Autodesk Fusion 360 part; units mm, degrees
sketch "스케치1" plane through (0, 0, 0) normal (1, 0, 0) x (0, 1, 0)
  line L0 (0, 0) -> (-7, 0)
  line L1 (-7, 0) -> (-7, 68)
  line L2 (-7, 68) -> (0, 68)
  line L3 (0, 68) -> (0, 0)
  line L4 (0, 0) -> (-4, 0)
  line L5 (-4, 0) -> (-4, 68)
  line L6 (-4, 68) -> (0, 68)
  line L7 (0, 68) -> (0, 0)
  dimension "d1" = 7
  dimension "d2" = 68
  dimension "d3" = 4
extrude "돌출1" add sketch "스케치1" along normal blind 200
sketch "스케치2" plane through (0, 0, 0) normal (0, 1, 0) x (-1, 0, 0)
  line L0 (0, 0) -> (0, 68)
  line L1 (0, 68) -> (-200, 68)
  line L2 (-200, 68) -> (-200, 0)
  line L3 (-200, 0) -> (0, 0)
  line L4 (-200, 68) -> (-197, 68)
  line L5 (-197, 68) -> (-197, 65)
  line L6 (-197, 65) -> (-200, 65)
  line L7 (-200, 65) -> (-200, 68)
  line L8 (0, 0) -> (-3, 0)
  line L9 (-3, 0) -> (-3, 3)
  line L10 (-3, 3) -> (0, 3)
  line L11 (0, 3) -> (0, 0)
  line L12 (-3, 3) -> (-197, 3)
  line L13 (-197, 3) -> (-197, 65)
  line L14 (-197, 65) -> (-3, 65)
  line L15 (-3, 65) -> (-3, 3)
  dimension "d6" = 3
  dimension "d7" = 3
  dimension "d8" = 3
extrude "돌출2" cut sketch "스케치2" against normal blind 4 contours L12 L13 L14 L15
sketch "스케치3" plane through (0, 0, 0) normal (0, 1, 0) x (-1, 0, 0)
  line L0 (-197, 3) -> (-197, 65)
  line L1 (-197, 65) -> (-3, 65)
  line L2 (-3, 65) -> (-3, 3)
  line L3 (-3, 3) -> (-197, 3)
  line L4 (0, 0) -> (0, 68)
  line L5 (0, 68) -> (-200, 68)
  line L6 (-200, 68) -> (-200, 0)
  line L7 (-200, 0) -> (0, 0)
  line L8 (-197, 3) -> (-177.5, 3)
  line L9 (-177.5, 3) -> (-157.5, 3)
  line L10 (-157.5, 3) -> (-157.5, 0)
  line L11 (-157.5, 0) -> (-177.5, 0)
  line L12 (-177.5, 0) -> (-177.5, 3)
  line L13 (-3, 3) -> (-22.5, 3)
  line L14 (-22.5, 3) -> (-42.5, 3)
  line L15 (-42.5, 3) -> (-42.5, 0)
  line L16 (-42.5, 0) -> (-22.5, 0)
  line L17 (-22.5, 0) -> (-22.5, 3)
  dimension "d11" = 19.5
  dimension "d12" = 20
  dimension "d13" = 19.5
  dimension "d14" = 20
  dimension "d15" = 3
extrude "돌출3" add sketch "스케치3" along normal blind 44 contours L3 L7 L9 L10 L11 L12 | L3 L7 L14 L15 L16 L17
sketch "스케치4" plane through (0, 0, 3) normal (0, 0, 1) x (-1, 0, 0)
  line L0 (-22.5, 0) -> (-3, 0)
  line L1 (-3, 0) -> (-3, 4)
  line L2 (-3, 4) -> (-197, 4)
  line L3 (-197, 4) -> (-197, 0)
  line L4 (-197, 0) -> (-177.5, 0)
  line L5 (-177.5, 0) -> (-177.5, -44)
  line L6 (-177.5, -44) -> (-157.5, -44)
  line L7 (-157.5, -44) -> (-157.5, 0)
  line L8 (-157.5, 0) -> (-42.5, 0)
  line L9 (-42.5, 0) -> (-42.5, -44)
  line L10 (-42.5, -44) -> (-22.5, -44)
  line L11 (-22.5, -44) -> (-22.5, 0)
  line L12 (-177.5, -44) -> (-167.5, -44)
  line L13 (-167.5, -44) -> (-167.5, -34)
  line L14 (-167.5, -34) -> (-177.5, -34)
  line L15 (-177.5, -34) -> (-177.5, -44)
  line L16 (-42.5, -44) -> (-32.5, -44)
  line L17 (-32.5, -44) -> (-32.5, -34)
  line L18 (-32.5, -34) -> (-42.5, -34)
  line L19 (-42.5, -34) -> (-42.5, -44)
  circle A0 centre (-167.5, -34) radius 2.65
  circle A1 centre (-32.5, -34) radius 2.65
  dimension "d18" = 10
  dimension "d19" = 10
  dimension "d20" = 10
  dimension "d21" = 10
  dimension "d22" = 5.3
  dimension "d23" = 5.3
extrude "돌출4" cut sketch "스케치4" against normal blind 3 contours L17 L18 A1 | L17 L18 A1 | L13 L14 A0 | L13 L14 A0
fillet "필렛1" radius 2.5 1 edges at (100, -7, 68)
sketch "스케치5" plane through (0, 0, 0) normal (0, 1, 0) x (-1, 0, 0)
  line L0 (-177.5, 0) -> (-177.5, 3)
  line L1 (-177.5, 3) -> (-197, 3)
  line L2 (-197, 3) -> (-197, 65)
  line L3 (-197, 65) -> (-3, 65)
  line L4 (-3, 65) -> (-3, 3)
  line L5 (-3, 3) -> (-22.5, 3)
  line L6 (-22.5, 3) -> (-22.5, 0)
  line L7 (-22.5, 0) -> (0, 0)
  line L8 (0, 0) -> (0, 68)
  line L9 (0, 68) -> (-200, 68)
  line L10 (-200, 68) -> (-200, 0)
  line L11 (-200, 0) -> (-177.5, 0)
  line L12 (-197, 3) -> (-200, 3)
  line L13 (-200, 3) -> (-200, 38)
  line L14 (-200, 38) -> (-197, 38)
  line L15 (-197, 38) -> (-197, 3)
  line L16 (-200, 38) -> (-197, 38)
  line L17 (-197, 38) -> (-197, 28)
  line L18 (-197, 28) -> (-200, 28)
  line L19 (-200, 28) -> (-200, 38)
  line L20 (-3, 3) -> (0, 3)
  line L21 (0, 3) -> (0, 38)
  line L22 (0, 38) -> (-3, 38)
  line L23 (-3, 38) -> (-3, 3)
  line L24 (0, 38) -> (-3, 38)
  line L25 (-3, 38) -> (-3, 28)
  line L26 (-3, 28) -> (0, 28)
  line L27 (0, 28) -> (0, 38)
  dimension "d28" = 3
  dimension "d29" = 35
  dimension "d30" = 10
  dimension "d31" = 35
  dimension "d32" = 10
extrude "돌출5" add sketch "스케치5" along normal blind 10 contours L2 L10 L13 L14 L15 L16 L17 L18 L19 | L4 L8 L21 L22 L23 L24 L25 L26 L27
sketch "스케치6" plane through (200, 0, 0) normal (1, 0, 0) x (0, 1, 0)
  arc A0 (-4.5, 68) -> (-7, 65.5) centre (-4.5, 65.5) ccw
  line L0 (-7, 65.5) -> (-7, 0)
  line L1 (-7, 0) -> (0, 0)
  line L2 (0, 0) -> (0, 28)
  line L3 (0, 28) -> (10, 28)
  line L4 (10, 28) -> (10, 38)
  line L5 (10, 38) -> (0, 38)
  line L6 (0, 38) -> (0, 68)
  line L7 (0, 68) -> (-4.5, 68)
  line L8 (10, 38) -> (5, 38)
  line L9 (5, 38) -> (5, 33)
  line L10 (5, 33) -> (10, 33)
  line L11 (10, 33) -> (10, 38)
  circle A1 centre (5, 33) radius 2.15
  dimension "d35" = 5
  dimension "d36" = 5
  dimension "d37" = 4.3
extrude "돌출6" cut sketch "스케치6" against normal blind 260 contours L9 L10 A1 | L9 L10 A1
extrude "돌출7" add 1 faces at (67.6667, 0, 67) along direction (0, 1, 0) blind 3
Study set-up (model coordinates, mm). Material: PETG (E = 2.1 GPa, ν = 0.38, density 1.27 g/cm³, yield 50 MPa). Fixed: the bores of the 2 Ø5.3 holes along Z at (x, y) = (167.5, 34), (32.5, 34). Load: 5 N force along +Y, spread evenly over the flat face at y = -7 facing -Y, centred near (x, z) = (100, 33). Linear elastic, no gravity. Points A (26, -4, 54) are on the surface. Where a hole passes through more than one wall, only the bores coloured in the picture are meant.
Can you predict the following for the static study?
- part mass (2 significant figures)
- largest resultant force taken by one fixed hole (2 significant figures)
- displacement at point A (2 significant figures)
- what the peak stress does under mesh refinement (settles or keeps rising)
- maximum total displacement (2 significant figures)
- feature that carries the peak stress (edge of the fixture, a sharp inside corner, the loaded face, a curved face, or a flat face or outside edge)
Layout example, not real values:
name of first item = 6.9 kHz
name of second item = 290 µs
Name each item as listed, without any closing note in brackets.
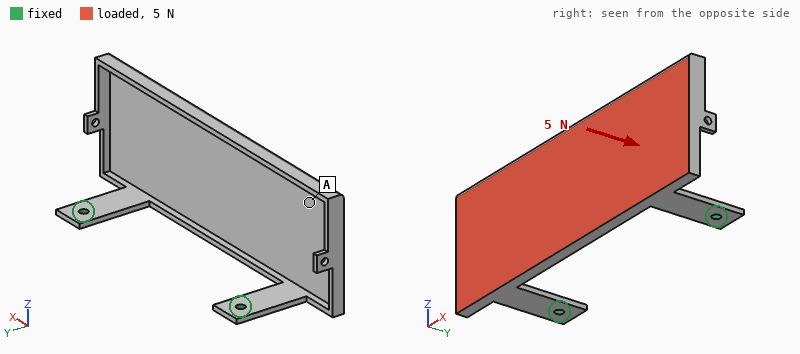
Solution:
part mass = 70 g
largest resultant force taken by one fixed hole = 2.6 N
displacement at point A = 1.8 mm
what the peak stress does under mesh refinement = keeps rising
maximum total displacement = 2.3 mm
feature that carries the peak stress = edge of the fixture
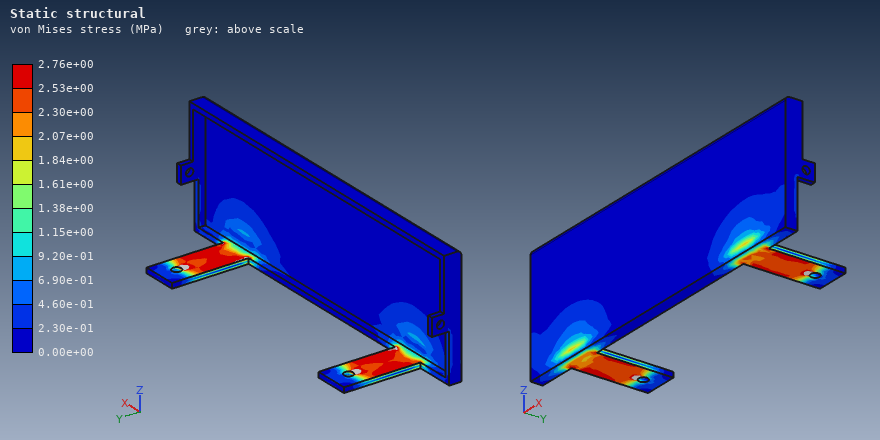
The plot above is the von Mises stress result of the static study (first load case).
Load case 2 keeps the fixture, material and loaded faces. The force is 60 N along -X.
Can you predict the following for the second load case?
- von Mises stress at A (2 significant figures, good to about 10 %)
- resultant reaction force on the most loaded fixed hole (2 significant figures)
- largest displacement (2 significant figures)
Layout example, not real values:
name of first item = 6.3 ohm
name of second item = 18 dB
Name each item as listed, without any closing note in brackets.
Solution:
von Mises stress at A = 1.1 MPa
resultant reaction force on the most loaded fixed hole = 33 N
largest displacement = 2.3 mm
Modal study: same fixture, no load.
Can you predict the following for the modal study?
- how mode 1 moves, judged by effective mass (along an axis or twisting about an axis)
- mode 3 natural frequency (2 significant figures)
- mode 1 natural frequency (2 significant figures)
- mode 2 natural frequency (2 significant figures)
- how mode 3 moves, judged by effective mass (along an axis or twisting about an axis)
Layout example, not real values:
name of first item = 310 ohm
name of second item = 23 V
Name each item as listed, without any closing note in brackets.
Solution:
how mode 1 moves, judged by effective mass = along Y
mode 3 natural frequency = 120 Hz
mode 1 natural frequency = 31 Hz
mode 2 natural frequency = 77 Hz
how mode 3 moves, judged by effective mass = along Z
